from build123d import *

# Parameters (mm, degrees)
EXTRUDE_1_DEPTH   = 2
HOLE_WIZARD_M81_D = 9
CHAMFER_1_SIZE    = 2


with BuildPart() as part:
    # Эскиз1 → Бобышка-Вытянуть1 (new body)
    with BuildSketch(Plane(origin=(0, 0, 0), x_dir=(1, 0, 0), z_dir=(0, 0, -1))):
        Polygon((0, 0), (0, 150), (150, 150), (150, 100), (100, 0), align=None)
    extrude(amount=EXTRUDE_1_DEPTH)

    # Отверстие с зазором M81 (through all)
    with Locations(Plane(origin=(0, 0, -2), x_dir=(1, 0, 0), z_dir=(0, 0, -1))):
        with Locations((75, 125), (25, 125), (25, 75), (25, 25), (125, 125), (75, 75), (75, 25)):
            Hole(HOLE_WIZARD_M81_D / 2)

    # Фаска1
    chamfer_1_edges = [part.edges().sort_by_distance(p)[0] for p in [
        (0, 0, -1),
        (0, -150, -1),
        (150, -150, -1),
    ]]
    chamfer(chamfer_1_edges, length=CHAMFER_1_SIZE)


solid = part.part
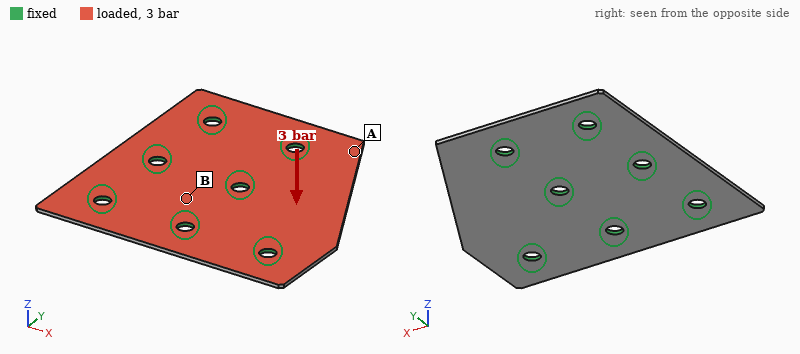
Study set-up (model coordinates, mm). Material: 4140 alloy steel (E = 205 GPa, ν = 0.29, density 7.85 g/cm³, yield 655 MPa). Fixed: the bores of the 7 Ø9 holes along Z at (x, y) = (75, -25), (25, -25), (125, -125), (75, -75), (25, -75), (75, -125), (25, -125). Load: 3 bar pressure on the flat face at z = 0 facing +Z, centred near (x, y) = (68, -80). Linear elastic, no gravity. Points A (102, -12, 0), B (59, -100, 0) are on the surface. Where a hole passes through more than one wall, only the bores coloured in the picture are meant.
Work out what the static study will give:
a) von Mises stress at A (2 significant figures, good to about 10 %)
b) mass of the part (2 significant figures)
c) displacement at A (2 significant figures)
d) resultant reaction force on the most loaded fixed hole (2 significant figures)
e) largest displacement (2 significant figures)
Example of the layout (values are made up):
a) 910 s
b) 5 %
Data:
a) 99 MPa
b) 310 g
c) 0.32 mm
d) 1.1 kN
e) 0.98 mm
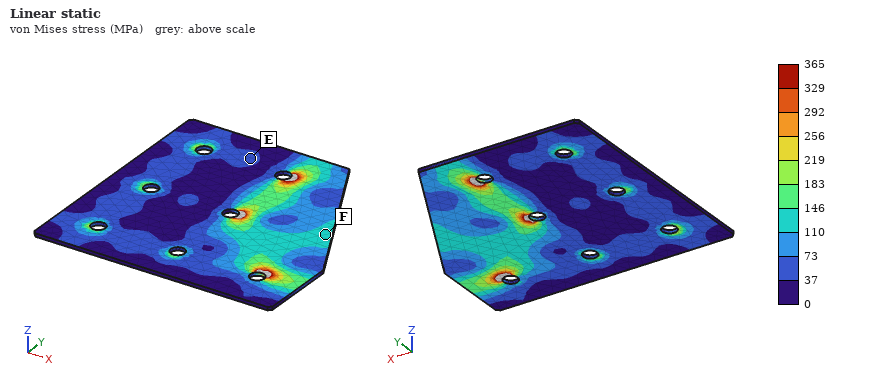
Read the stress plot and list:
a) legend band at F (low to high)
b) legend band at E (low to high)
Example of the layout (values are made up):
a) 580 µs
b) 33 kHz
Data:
a) 110 to 146 MPa
b) 37 to 73 MPa
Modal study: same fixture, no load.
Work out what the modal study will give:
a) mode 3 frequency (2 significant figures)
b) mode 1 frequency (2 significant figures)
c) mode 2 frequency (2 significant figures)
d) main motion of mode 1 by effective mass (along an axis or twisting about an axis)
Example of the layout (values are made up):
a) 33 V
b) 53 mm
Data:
a) 2500 Hz
b) 950 Hz
c) 1800 Hz
d) along Z
